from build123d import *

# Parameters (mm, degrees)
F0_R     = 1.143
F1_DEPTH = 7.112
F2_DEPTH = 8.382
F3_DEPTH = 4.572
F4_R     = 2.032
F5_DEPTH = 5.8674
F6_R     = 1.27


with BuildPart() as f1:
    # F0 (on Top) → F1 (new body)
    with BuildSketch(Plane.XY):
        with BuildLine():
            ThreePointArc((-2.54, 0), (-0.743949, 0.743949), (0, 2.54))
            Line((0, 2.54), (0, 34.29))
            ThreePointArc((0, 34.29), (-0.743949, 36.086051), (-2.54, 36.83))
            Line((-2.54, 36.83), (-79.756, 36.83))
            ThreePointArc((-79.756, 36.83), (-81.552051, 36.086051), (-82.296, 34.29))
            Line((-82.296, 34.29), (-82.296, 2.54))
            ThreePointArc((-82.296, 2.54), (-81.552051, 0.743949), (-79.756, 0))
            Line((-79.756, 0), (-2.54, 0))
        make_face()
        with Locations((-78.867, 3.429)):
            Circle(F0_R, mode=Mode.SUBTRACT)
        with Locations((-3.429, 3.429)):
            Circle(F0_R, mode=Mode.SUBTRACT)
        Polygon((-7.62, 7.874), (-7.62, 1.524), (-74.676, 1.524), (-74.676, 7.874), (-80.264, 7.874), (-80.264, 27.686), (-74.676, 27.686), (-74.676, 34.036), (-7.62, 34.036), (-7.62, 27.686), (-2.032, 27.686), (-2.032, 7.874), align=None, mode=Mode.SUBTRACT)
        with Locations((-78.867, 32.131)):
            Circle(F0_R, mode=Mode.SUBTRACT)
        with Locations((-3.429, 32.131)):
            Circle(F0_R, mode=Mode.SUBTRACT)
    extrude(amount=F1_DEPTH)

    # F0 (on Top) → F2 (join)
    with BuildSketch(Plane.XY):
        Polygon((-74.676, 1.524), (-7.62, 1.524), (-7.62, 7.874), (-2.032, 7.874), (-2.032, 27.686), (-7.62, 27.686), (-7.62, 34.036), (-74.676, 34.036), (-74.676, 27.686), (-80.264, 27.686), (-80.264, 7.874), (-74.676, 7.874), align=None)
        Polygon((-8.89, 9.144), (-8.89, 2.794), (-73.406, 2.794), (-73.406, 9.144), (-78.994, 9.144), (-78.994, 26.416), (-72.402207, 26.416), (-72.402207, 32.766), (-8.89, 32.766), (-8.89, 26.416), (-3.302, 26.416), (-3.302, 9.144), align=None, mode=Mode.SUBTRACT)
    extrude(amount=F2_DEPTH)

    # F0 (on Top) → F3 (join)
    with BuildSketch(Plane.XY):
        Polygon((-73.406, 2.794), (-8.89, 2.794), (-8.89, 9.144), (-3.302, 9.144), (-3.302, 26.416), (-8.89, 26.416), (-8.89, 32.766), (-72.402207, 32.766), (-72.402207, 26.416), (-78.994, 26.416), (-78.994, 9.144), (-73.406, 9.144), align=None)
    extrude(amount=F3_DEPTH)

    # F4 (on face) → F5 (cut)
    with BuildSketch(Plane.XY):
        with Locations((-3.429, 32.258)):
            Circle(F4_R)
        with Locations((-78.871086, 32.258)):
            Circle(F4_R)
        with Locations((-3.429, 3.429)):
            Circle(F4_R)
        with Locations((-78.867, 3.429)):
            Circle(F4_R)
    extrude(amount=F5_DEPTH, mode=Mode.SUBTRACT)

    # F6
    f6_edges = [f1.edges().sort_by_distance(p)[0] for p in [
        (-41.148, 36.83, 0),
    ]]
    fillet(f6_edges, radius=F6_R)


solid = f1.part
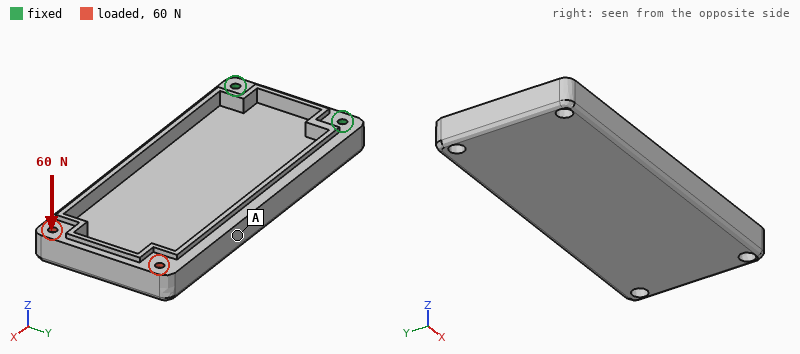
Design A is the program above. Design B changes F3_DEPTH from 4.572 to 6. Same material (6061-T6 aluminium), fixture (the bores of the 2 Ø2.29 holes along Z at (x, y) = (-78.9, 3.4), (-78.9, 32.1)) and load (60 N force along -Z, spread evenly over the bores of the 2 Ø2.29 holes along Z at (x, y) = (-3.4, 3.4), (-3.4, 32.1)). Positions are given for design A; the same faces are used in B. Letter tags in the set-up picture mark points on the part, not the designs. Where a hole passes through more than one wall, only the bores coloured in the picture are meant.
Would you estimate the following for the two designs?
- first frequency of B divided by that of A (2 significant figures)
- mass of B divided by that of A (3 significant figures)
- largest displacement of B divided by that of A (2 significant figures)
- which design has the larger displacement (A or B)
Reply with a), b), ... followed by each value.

a) 0.95
b) 1.19
c) 0.92
d) A
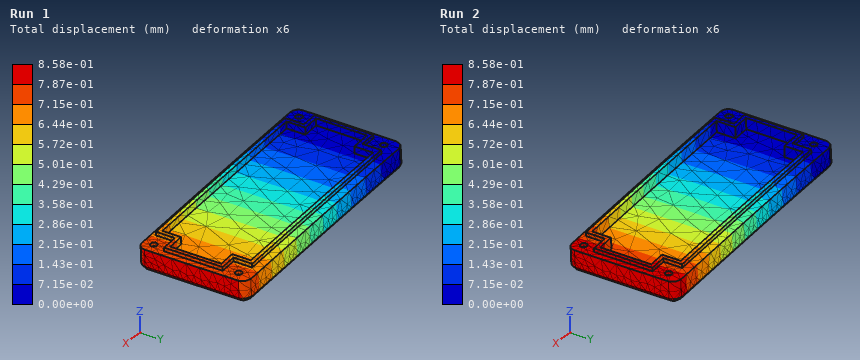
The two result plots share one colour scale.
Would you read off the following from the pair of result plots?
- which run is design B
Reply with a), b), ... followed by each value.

a) Run 1
